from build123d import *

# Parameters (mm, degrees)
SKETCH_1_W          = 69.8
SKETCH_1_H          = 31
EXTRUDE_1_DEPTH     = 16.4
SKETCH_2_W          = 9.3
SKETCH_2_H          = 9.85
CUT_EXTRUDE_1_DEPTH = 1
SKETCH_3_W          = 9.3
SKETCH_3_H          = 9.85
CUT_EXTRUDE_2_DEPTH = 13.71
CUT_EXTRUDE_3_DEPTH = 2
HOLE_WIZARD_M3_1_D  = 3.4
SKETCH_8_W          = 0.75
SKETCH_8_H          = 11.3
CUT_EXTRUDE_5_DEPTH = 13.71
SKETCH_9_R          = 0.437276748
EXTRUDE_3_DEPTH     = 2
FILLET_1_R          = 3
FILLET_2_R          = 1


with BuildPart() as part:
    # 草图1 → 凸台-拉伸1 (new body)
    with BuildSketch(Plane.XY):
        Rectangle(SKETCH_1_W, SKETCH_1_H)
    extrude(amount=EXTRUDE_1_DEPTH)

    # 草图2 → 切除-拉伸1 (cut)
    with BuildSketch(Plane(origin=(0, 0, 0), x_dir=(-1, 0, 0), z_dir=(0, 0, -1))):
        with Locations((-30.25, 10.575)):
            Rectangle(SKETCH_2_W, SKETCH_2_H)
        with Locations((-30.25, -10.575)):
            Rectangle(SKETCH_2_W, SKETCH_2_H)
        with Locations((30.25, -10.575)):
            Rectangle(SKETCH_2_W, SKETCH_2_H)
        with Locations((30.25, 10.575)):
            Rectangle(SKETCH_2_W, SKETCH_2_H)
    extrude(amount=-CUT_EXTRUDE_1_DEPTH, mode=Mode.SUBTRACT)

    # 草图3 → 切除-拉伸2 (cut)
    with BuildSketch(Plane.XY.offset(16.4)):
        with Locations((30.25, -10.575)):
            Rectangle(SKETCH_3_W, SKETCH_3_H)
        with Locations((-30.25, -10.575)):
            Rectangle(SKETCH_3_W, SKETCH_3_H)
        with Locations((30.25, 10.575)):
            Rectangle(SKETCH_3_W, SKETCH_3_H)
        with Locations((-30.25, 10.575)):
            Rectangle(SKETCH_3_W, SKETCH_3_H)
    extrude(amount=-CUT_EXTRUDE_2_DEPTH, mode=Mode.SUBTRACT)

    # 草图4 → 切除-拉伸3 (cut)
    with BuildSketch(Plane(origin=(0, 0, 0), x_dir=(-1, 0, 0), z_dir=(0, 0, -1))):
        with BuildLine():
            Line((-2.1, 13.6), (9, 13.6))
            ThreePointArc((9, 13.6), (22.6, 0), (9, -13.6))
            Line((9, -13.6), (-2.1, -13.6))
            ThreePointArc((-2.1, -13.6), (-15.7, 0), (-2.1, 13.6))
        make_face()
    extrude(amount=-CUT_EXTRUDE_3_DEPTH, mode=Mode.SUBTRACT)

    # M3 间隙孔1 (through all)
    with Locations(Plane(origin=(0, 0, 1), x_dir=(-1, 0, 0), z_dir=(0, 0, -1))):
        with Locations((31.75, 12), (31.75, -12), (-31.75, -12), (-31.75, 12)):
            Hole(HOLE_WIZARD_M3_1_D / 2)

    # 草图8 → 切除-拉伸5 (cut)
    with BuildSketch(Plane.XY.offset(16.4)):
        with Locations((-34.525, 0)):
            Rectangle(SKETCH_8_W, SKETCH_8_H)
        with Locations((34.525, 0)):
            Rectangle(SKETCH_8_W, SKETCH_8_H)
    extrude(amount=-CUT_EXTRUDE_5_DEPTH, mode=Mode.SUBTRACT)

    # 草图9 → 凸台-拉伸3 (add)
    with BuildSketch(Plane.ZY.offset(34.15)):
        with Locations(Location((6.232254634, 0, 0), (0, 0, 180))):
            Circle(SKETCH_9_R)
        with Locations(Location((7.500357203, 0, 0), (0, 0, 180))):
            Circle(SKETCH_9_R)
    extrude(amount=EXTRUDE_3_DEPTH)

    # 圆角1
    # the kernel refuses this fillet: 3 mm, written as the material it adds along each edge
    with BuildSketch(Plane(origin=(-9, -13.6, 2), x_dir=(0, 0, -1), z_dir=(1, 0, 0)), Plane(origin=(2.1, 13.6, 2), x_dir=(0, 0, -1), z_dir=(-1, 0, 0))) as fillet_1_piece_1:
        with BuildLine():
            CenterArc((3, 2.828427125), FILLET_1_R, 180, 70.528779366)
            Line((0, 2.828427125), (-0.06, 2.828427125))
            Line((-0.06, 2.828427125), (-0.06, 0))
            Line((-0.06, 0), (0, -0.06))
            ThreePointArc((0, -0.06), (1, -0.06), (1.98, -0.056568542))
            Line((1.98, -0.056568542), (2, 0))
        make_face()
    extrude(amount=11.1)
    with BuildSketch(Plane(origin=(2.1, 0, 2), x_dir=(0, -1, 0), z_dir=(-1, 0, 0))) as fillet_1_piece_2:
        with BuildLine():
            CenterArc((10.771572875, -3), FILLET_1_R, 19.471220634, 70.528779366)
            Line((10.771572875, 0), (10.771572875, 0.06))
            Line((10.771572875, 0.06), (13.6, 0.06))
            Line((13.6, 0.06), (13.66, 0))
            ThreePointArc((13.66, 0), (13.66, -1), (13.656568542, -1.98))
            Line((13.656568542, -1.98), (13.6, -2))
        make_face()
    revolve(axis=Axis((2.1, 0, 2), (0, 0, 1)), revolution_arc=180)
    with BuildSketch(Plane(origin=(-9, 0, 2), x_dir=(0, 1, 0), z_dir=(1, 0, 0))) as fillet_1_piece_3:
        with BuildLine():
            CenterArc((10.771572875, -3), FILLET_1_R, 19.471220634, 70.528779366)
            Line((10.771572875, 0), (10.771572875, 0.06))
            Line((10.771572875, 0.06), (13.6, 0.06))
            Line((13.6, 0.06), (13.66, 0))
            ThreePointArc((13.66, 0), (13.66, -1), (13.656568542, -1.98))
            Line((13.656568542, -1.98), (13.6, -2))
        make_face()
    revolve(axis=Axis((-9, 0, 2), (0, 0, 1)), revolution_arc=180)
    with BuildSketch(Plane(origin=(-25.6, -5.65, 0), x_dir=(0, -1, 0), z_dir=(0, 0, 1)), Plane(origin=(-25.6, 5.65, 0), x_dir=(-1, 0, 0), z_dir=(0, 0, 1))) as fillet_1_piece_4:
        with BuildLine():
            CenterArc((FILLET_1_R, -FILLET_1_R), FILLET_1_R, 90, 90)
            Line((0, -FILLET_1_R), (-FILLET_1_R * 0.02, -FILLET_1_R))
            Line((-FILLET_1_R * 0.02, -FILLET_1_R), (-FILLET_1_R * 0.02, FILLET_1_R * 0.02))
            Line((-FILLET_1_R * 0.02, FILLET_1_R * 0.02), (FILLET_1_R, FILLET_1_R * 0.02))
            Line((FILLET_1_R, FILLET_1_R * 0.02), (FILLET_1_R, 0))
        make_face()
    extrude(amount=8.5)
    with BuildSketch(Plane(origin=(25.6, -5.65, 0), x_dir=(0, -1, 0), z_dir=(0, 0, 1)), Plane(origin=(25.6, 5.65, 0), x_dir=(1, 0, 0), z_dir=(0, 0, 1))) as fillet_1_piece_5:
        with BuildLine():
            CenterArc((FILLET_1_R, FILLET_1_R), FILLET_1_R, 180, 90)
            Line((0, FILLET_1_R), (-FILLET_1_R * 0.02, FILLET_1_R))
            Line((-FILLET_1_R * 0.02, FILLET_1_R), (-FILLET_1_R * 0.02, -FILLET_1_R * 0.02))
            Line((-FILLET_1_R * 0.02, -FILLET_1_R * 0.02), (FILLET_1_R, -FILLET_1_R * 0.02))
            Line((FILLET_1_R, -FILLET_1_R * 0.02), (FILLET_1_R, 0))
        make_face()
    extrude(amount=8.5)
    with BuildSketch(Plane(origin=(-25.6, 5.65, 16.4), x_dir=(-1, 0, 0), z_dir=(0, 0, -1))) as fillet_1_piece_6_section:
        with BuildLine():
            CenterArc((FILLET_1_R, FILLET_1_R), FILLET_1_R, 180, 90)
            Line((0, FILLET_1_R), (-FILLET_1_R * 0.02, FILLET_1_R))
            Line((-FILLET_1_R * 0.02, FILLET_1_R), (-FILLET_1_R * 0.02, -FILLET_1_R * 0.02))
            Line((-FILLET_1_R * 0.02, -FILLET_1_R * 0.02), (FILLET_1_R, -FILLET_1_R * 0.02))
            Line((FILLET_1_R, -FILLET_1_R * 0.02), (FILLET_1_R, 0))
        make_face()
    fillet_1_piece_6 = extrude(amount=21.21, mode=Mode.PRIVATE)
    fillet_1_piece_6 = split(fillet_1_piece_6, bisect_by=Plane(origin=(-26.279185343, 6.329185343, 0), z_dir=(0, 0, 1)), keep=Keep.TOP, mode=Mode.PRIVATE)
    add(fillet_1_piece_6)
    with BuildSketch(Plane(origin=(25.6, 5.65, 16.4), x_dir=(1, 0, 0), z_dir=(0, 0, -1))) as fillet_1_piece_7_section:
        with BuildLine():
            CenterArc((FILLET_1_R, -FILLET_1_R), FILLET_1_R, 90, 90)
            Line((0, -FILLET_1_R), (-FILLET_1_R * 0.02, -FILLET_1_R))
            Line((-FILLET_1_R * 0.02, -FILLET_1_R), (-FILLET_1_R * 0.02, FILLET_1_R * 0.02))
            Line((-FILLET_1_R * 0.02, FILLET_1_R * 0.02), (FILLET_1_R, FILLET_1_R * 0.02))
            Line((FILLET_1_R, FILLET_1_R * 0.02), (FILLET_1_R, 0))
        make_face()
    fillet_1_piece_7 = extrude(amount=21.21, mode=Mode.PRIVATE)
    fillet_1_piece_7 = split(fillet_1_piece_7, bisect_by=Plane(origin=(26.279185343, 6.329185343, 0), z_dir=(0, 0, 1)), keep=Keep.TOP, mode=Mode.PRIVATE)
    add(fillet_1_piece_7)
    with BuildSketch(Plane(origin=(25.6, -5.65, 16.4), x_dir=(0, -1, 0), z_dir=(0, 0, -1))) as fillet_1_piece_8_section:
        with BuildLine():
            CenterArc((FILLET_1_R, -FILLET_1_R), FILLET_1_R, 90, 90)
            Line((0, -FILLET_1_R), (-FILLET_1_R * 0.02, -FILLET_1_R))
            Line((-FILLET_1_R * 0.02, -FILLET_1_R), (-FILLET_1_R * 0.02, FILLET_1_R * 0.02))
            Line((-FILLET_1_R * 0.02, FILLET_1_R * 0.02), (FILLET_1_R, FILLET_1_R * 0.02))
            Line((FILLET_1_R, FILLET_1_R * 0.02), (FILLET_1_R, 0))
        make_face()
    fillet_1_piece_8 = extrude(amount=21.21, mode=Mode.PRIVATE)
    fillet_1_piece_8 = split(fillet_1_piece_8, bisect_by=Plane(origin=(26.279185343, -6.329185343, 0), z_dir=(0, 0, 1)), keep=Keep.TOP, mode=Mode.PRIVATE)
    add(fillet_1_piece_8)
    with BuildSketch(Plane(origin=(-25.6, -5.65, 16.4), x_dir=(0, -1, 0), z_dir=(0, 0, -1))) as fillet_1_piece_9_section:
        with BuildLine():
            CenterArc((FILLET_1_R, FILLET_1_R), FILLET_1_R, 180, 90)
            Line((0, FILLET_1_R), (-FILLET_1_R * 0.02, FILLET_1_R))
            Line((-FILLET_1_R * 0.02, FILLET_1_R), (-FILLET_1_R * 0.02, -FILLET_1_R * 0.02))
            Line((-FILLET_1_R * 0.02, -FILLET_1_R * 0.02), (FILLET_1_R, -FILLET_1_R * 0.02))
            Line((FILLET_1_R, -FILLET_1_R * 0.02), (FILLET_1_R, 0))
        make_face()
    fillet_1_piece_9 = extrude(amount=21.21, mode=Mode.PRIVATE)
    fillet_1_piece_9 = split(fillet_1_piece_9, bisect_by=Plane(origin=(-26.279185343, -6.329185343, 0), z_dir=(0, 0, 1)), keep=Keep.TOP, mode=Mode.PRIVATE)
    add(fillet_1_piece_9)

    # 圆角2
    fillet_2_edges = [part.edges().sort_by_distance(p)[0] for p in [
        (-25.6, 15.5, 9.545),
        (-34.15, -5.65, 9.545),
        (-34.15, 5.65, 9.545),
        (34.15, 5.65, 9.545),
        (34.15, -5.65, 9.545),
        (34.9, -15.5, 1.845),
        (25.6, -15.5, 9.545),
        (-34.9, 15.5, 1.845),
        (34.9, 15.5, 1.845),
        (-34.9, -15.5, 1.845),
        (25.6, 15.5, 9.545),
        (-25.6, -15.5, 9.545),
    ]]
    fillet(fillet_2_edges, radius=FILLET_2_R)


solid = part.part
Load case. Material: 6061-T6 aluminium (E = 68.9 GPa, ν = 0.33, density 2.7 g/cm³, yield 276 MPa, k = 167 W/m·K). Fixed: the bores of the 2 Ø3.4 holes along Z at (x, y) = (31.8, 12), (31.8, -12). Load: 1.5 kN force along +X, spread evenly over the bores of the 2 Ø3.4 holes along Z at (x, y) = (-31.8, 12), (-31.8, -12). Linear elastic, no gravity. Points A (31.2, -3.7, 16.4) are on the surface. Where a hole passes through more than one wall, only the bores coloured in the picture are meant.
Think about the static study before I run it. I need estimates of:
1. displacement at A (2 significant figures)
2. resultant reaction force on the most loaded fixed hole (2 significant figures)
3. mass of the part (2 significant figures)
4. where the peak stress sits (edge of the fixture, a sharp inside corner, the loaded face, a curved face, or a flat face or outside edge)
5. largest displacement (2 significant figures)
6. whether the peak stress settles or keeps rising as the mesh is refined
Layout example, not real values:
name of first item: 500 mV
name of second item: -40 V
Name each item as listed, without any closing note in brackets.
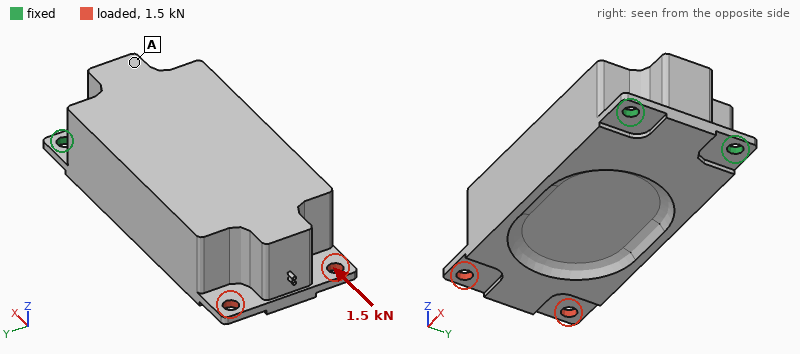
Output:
displacement at A: 5.9 µm
resultant reaction force on the most loaded fixed hole: 760 N
mass of the part: 76 g
where the peak stress sits: a sharp inside corner
largest displacement: 35 µm
whether the peak stress settles or keeps rising as the mesh is refined: keeps rising
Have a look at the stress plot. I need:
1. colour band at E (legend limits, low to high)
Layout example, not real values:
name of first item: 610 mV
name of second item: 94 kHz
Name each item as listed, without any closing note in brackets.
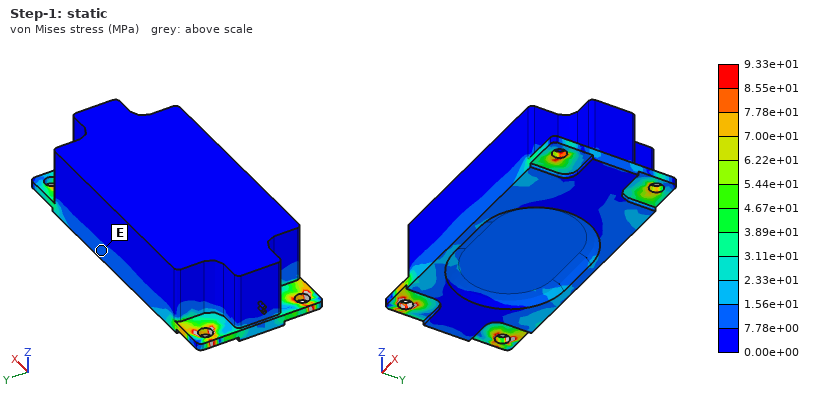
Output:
colour band at E: 7.78e+00 to 1.56e+01 MPa
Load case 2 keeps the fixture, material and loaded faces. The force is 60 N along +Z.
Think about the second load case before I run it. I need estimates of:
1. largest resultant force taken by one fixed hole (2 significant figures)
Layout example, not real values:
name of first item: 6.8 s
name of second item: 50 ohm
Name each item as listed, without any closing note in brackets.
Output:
largest resultant force taken by one fixed hole: 37 N
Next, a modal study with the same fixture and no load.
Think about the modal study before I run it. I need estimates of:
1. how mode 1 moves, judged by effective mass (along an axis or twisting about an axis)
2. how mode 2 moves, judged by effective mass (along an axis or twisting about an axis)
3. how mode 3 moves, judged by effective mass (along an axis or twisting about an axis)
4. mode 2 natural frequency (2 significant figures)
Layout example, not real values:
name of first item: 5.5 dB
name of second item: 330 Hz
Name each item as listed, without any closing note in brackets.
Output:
how mode 1 moves, judged by effective mass: along Z
how mode 2 moves, judged by effective mass: along Y
how mode 3 moves, judged by effective mass: twisting about X
mode 2 natural frequency: 2500 Hz
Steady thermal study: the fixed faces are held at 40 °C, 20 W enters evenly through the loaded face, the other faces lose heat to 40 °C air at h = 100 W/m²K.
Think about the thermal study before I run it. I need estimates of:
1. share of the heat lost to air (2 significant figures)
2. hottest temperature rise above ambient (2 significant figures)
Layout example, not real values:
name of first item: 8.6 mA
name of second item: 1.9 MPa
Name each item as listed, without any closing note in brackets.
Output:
share of the heat lost to air: 51 %
hottest temperature rise above ambient: 46 K
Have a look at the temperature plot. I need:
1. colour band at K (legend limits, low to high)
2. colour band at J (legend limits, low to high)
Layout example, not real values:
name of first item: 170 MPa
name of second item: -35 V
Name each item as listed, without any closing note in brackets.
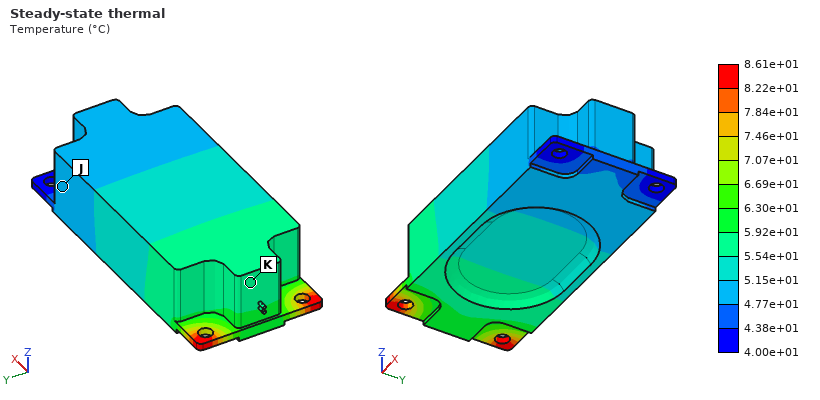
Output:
colour band at K: 5.54e+01 to 5.92e+01 °C
colour band at J: 4.77e+01 to 5.15e+01 °C
